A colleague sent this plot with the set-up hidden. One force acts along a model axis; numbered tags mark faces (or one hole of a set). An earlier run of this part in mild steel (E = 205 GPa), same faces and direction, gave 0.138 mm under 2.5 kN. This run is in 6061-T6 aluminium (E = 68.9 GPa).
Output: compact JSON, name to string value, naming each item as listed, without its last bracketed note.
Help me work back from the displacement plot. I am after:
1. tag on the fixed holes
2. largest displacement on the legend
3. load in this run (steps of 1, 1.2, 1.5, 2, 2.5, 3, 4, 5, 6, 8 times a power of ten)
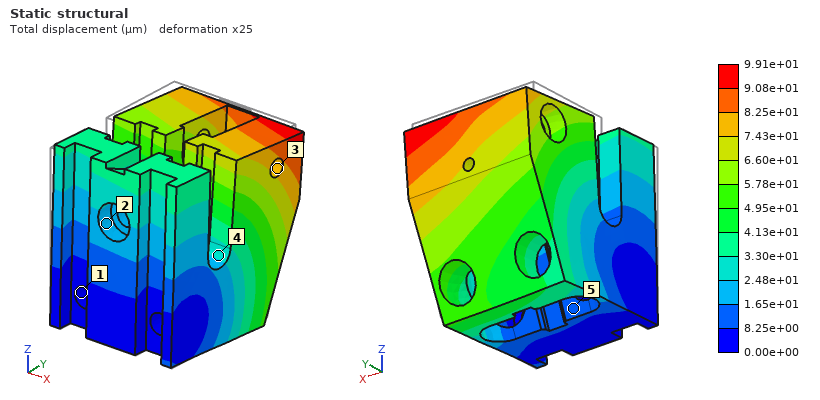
{"tag on the fixed holes": "1", "largest displacement on the legend": "9.91e+01 µm", "load in this run": "600 N"}
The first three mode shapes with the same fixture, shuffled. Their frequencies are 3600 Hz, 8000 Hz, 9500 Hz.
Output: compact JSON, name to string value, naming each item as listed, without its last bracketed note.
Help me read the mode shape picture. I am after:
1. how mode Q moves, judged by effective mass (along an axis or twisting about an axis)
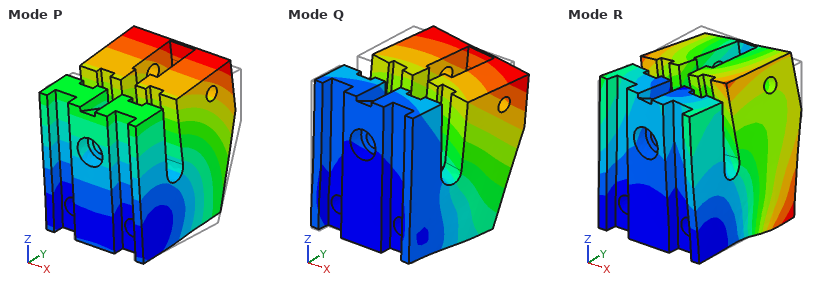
{"how mode Q moves, judged by effective mass": "along X"}
